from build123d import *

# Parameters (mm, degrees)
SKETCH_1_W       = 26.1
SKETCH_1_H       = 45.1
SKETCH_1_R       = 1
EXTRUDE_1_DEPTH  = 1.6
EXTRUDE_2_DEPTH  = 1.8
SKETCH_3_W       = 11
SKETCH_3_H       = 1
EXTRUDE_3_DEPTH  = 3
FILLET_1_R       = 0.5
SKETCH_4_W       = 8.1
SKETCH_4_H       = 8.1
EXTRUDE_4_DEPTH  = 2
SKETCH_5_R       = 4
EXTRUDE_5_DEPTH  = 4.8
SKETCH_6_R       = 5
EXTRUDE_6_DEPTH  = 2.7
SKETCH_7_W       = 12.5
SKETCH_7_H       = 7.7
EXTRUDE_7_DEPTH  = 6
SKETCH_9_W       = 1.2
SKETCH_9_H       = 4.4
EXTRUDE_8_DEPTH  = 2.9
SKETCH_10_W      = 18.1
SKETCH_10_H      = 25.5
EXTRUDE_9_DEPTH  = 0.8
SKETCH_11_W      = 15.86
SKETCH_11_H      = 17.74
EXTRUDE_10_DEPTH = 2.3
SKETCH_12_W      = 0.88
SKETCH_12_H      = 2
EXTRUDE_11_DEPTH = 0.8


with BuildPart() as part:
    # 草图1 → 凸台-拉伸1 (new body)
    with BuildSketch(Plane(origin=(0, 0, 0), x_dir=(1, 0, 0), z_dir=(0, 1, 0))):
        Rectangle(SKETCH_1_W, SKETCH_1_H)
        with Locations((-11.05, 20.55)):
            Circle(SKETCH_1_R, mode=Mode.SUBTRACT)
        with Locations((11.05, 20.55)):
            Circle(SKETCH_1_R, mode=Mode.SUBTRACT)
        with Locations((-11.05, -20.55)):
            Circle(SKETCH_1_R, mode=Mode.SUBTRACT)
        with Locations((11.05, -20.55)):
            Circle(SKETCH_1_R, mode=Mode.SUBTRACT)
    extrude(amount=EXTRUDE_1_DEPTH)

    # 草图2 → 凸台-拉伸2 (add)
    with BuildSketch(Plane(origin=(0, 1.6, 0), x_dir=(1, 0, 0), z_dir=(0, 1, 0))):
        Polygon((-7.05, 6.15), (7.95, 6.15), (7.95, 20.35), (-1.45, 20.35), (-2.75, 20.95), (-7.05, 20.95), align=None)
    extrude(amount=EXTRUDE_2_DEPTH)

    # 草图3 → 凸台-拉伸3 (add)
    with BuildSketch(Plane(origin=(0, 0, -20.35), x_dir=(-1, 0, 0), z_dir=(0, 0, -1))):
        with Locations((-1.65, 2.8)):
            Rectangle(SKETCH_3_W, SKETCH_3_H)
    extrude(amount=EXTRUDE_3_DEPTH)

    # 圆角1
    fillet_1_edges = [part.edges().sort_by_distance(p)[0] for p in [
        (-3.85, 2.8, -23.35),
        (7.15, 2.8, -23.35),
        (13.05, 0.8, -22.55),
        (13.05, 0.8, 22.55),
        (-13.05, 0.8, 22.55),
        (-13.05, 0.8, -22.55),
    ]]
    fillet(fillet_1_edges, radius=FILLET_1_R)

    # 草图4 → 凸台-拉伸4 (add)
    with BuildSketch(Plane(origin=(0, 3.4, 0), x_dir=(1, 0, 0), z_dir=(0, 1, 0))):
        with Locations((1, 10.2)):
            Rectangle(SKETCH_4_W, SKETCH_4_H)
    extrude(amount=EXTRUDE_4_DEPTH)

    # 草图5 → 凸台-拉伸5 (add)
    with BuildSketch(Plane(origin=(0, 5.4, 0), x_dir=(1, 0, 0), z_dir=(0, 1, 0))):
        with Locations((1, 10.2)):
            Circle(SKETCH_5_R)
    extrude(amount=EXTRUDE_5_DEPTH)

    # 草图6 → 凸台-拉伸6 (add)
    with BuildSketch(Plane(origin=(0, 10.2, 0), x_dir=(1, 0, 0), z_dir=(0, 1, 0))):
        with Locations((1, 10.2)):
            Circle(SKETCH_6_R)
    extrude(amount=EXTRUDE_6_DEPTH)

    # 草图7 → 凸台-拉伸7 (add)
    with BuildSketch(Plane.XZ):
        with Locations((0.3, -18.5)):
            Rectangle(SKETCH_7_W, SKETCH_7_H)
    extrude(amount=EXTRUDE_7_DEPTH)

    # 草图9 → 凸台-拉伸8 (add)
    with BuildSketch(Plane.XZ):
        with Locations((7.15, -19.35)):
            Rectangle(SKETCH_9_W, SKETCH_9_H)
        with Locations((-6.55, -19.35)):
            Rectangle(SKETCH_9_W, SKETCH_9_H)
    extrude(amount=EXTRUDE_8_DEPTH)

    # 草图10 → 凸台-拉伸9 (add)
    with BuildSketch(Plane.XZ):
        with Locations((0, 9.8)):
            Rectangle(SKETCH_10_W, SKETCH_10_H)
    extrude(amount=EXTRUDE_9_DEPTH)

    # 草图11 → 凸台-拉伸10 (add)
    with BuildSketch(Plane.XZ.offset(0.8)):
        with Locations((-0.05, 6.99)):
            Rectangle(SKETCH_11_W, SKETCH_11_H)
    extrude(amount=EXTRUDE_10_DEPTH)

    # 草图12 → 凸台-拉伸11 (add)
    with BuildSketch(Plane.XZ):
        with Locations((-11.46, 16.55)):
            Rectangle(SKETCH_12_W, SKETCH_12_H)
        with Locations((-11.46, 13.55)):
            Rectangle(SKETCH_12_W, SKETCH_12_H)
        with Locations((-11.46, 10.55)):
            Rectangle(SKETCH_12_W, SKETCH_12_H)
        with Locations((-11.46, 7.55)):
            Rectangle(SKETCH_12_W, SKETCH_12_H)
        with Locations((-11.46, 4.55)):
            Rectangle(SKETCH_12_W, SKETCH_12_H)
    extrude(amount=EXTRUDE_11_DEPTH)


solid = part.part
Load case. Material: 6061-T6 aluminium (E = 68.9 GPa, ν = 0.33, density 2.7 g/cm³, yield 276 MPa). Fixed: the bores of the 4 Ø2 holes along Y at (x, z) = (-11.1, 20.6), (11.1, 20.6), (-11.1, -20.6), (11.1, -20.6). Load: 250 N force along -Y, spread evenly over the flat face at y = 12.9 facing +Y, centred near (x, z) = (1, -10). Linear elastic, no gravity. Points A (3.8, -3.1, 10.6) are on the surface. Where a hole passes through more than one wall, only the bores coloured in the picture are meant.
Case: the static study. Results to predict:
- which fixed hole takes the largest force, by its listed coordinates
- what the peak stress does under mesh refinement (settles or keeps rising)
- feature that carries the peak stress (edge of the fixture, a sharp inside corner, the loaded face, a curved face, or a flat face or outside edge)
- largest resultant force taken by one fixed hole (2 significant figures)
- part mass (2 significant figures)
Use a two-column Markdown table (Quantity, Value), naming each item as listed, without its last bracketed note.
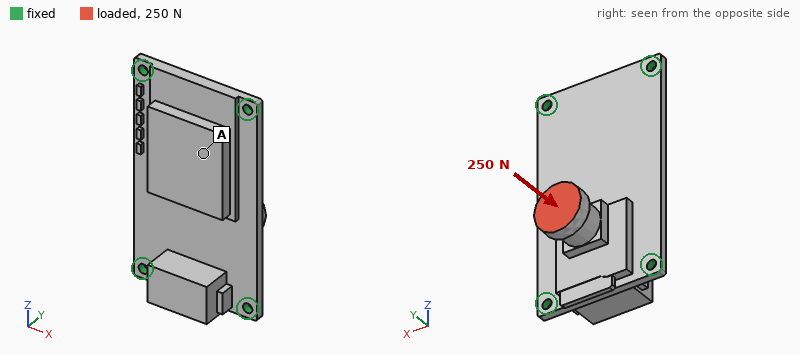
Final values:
| Quantity | Value |
|---|---|
| which fixed hole takes the largest force, by its listed coordinates | (11.1, -20.6) |
| what the peak stress does under mesh refinement | keeps rising |
| feature that carries the peak stress | edge of the fixture |
| largest resultant force taken by one fixed hole | 110 N |
| part mass | 12 g |
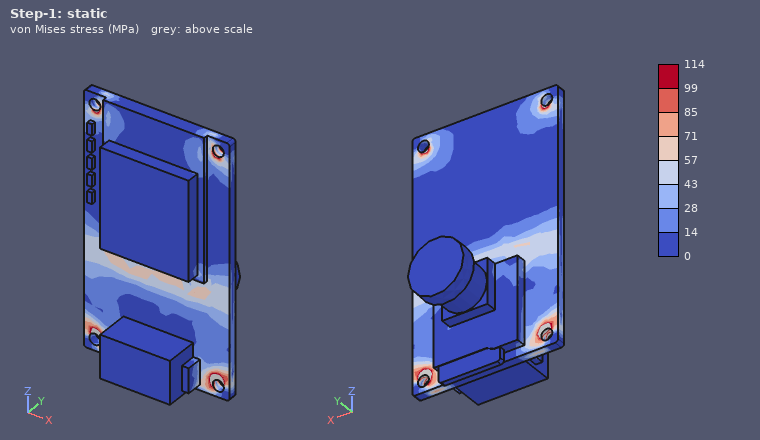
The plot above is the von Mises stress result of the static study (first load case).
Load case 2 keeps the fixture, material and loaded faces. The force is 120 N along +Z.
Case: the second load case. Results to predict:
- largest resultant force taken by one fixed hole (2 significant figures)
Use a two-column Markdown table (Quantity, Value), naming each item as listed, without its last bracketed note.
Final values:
| Quantity | Value |
|---|---|
| largest resultant force taken by one fixed hole | 53 N |
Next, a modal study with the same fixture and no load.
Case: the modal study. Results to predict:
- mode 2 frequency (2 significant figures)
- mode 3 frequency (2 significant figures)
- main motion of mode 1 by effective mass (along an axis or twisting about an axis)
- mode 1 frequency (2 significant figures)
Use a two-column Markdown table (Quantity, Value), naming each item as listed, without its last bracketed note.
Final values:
| Quantity | Value |
|---|---|
| mode 2 frequency | 12 kHz |
| mode 3 frequency | 15 kHz |
| main motion of mode 1 by effective mass | along Y |
| mode 1 frequency | 3700 Hz |
